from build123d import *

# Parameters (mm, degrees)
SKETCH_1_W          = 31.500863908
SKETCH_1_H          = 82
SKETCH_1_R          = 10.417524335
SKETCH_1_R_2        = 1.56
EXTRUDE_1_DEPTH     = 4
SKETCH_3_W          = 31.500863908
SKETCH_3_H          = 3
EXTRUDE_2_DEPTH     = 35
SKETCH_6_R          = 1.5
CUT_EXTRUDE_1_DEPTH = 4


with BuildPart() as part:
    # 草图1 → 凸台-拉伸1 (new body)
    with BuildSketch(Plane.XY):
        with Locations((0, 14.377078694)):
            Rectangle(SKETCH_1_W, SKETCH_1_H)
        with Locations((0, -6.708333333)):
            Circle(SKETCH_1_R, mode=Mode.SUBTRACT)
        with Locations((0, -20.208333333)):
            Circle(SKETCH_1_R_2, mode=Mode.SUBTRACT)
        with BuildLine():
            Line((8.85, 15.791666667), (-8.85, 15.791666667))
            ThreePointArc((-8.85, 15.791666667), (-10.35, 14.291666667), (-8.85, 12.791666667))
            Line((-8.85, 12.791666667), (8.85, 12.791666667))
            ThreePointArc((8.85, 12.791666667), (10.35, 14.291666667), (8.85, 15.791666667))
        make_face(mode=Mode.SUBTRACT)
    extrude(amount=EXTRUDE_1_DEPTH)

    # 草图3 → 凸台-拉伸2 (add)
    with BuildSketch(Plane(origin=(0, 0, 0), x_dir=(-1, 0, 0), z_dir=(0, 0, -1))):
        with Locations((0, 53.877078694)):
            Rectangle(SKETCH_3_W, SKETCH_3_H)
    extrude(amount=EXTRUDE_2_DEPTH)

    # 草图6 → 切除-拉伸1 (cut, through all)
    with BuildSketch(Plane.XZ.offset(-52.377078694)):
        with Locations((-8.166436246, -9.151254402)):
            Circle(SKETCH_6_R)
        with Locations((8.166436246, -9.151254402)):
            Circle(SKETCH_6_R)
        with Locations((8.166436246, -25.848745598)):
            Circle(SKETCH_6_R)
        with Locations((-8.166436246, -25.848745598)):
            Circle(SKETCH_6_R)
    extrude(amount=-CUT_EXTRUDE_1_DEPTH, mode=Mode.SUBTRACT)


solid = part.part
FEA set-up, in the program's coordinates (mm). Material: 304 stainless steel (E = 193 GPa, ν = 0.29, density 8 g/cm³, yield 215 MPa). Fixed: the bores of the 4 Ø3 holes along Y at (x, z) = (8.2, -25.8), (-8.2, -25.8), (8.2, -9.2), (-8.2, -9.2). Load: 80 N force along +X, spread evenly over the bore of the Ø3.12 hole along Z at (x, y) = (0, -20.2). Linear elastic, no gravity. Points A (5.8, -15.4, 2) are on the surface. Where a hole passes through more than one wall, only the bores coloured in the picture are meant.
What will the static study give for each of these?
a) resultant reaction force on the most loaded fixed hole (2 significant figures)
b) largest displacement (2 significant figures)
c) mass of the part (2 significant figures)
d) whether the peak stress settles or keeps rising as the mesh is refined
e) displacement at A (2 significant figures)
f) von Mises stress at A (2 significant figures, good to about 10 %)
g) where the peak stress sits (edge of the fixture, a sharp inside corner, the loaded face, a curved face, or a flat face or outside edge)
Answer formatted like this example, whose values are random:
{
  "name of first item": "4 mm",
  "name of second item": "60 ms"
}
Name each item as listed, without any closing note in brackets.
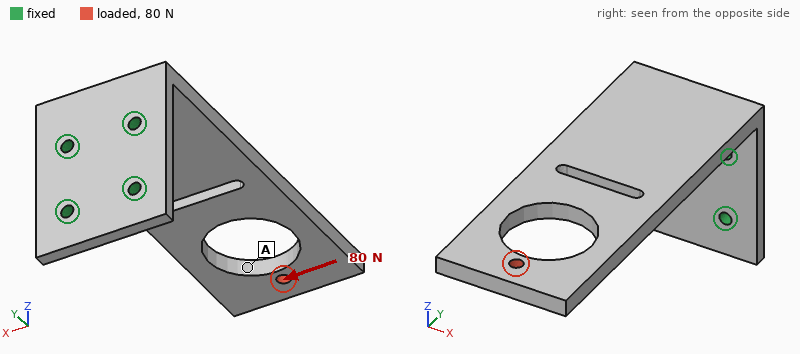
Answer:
{
  "resultant reaction force on the most loaded fixed hole": "320 N",
  "largest displacement": "79 µm",
  "mass of the part": "95 g",
  "whether the peak stress settles or keeps rising as the mesh is refined": "keeps rising",
  "displacement at A": "66 µm",
  "von Mises stress at A": "7.6 MPa",
  "where the peak stress sits": "edge of the fixture"
}
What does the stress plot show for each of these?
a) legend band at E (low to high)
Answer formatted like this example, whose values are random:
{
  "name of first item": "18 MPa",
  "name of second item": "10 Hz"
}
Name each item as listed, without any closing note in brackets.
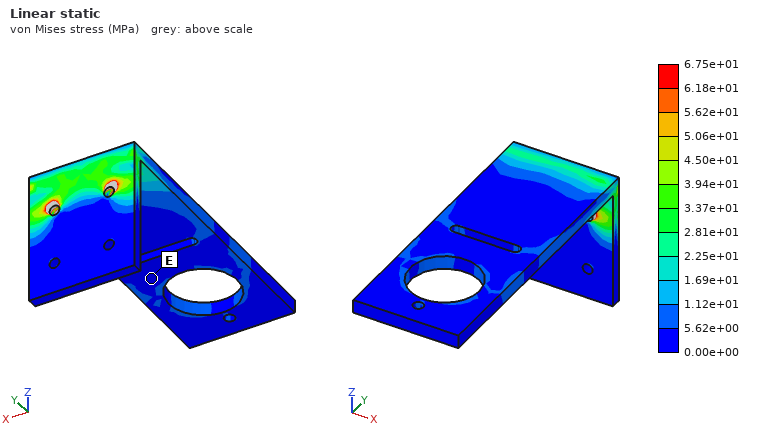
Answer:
{
  "legend band at E": "0.00e+00 to 5.62e+00 MPa"
}
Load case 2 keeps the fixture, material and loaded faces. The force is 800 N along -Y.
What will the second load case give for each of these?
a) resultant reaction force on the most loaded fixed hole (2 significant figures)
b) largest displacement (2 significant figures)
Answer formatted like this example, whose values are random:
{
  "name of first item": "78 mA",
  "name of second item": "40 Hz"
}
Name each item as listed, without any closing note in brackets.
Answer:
{
  "resultant reaction force on the most loaded fixed hole": "460 N",
  "largest displacement": "0.29 mm"
}
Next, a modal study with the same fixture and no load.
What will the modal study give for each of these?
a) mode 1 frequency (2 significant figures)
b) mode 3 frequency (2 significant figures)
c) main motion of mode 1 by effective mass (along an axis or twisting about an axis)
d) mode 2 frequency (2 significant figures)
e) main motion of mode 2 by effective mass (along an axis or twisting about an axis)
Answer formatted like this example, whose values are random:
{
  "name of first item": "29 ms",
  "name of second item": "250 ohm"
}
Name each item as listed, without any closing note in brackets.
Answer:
{
  "mode 1 frequency": "380 Hz",
  "mode 3 frequency": "1900 Hz",
  "main motion of mode 1 by effective mass": "along Z",
  "mode 2 frequency": "1100 Hz",
  "main motion of mode 2 by effective mass": "along X"
}
